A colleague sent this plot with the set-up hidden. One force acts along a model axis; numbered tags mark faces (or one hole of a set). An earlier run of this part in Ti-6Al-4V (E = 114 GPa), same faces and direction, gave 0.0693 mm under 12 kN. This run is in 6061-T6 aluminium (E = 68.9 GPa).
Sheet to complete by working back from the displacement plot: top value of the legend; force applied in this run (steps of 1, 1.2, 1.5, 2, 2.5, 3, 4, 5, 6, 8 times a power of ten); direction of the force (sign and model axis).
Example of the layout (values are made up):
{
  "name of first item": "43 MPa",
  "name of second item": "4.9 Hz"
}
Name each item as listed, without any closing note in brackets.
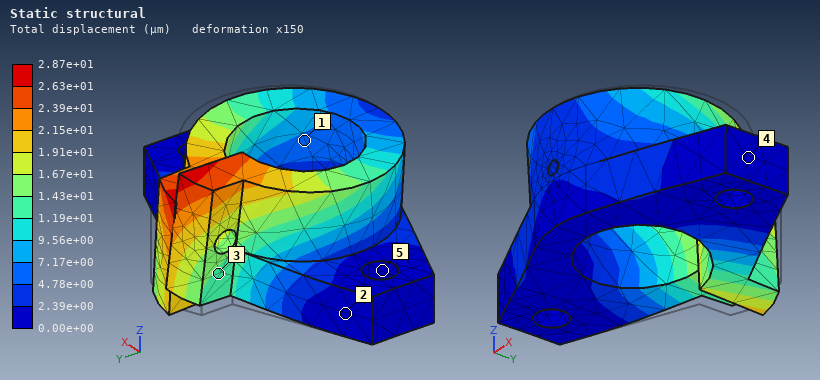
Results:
{
  "top value of the legend": "2.87e+01 µm",
  "force applied in this run": "3 kN",
  "direction of the force": "-X"
}
